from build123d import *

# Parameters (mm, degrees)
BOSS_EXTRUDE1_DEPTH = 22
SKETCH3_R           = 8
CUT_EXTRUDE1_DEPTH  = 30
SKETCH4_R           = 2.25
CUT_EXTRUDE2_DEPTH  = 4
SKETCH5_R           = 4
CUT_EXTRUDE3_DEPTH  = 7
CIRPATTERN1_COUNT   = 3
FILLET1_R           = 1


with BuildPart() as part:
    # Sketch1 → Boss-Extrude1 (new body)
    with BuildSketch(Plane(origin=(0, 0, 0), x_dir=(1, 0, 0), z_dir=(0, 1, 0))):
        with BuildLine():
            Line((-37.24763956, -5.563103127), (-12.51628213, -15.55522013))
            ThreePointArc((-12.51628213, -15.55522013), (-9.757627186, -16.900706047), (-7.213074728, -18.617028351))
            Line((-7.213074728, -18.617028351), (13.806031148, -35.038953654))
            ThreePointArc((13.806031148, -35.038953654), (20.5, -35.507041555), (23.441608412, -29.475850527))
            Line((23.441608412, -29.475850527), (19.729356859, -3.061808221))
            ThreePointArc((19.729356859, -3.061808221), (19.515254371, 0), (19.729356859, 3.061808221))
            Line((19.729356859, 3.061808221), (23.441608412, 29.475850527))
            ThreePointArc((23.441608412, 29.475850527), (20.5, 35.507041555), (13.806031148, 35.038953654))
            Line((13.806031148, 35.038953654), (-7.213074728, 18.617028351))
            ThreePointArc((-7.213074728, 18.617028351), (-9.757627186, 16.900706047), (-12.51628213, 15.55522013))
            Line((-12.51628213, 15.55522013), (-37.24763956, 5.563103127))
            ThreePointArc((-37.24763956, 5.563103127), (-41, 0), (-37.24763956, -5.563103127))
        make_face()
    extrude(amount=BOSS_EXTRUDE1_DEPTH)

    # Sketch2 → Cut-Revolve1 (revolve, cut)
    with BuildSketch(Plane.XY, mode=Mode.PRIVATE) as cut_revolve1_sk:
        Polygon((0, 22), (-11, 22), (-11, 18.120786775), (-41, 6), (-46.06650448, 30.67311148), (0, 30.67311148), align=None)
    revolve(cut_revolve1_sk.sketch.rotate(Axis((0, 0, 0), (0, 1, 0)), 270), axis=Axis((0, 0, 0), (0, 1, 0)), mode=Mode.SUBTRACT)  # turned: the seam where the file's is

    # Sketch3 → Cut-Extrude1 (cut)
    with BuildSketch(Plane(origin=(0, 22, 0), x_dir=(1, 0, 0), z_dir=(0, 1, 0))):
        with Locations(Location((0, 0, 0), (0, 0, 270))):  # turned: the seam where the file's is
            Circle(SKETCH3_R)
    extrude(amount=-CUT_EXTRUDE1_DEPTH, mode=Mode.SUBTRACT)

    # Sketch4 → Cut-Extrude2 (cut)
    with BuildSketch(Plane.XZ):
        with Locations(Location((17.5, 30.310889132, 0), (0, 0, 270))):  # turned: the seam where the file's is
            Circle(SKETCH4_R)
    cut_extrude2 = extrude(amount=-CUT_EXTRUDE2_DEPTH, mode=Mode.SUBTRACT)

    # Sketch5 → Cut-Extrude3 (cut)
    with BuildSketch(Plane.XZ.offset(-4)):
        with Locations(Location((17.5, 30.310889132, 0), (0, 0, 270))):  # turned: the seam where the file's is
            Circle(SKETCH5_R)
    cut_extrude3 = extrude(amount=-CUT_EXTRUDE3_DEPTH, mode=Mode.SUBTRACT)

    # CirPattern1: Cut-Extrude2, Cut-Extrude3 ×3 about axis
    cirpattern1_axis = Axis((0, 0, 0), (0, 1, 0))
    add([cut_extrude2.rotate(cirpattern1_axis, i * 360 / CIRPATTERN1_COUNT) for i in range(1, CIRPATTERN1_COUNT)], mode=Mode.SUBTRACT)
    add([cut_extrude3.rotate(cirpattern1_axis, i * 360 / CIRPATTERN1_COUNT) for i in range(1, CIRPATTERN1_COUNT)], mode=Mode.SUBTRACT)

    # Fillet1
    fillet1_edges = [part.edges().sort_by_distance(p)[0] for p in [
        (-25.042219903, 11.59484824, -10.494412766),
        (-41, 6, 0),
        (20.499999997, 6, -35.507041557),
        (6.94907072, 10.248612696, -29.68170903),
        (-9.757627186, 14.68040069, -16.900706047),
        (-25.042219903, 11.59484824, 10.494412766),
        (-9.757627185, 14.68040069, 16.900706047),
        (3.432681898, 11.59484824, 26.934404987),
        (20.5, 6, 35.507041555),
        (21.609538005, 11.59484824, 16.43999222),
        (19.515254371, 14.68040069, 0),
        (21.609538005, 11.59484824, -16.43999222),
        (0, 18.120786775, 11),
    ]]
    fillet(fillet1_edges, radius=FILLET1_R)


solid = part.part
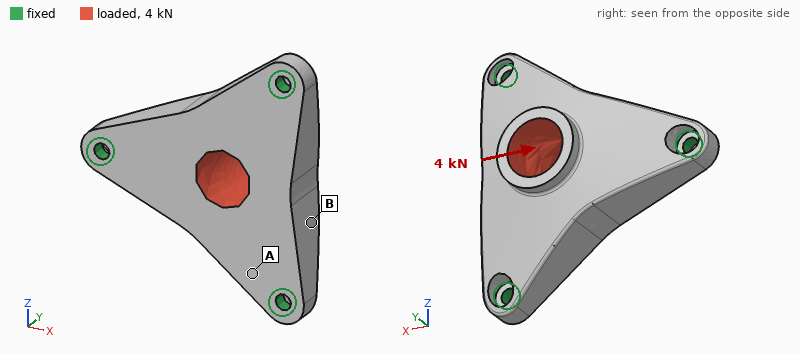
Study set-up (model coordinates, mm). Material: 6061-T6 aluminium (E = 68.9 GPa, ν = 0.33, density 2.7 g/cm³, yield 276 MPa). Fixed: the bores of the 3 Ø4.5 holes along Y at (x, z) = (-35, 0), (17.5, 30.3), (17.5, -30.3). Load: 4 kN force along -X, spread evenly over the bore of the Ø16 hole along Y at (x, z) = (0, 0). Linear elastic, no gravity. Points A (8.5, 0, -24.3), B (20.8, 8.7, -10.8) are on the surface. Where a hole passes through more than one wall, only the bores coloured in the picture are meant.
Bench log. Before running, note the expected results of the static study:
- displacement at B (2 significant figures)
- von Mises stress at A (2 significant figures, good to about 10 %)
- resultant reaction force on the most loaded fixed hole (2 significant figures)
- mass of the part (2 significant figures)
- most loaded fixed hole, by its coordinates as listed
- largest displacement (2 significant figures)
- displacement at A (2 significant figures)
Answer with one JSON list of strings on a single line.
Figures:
["8.2 µm", "12 MPa", "2.2 kN", "82 g", "(-35, 0)", "14 µm", "3.1 µm"]
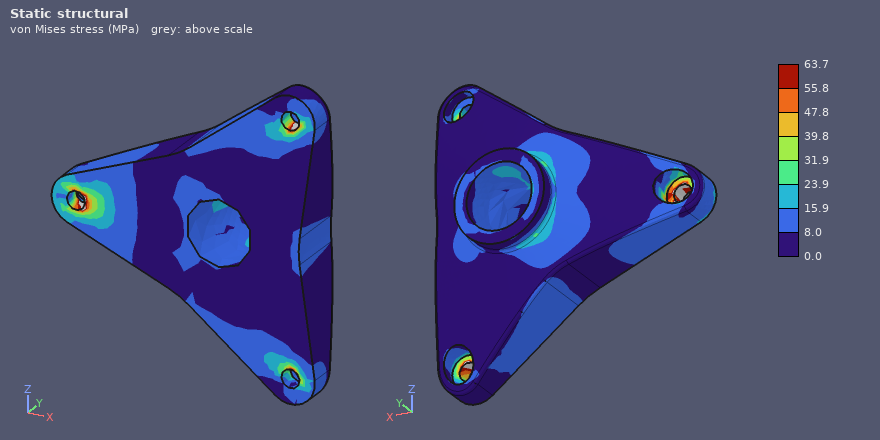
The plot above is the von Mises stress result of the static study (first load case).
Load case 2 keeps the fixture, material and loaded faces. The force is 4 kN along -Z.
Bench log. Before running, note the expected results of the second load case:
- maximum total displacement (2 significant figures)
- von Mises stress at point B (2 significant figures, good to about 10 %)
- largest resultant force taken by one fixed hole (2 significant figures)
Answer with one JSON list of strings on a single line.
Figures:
["13 µm", "10 MPa", "2.0 kN"]
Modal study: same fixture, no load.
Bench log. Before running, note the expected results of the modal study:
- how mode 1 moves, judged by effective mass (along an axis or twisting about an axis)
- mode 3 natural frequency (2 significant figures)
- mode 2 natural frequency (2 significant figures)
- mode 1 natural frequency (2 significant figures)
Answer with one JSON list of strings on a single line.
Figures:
["along Y", "15 kHz", "15 kHz", "9800 Hz"]
